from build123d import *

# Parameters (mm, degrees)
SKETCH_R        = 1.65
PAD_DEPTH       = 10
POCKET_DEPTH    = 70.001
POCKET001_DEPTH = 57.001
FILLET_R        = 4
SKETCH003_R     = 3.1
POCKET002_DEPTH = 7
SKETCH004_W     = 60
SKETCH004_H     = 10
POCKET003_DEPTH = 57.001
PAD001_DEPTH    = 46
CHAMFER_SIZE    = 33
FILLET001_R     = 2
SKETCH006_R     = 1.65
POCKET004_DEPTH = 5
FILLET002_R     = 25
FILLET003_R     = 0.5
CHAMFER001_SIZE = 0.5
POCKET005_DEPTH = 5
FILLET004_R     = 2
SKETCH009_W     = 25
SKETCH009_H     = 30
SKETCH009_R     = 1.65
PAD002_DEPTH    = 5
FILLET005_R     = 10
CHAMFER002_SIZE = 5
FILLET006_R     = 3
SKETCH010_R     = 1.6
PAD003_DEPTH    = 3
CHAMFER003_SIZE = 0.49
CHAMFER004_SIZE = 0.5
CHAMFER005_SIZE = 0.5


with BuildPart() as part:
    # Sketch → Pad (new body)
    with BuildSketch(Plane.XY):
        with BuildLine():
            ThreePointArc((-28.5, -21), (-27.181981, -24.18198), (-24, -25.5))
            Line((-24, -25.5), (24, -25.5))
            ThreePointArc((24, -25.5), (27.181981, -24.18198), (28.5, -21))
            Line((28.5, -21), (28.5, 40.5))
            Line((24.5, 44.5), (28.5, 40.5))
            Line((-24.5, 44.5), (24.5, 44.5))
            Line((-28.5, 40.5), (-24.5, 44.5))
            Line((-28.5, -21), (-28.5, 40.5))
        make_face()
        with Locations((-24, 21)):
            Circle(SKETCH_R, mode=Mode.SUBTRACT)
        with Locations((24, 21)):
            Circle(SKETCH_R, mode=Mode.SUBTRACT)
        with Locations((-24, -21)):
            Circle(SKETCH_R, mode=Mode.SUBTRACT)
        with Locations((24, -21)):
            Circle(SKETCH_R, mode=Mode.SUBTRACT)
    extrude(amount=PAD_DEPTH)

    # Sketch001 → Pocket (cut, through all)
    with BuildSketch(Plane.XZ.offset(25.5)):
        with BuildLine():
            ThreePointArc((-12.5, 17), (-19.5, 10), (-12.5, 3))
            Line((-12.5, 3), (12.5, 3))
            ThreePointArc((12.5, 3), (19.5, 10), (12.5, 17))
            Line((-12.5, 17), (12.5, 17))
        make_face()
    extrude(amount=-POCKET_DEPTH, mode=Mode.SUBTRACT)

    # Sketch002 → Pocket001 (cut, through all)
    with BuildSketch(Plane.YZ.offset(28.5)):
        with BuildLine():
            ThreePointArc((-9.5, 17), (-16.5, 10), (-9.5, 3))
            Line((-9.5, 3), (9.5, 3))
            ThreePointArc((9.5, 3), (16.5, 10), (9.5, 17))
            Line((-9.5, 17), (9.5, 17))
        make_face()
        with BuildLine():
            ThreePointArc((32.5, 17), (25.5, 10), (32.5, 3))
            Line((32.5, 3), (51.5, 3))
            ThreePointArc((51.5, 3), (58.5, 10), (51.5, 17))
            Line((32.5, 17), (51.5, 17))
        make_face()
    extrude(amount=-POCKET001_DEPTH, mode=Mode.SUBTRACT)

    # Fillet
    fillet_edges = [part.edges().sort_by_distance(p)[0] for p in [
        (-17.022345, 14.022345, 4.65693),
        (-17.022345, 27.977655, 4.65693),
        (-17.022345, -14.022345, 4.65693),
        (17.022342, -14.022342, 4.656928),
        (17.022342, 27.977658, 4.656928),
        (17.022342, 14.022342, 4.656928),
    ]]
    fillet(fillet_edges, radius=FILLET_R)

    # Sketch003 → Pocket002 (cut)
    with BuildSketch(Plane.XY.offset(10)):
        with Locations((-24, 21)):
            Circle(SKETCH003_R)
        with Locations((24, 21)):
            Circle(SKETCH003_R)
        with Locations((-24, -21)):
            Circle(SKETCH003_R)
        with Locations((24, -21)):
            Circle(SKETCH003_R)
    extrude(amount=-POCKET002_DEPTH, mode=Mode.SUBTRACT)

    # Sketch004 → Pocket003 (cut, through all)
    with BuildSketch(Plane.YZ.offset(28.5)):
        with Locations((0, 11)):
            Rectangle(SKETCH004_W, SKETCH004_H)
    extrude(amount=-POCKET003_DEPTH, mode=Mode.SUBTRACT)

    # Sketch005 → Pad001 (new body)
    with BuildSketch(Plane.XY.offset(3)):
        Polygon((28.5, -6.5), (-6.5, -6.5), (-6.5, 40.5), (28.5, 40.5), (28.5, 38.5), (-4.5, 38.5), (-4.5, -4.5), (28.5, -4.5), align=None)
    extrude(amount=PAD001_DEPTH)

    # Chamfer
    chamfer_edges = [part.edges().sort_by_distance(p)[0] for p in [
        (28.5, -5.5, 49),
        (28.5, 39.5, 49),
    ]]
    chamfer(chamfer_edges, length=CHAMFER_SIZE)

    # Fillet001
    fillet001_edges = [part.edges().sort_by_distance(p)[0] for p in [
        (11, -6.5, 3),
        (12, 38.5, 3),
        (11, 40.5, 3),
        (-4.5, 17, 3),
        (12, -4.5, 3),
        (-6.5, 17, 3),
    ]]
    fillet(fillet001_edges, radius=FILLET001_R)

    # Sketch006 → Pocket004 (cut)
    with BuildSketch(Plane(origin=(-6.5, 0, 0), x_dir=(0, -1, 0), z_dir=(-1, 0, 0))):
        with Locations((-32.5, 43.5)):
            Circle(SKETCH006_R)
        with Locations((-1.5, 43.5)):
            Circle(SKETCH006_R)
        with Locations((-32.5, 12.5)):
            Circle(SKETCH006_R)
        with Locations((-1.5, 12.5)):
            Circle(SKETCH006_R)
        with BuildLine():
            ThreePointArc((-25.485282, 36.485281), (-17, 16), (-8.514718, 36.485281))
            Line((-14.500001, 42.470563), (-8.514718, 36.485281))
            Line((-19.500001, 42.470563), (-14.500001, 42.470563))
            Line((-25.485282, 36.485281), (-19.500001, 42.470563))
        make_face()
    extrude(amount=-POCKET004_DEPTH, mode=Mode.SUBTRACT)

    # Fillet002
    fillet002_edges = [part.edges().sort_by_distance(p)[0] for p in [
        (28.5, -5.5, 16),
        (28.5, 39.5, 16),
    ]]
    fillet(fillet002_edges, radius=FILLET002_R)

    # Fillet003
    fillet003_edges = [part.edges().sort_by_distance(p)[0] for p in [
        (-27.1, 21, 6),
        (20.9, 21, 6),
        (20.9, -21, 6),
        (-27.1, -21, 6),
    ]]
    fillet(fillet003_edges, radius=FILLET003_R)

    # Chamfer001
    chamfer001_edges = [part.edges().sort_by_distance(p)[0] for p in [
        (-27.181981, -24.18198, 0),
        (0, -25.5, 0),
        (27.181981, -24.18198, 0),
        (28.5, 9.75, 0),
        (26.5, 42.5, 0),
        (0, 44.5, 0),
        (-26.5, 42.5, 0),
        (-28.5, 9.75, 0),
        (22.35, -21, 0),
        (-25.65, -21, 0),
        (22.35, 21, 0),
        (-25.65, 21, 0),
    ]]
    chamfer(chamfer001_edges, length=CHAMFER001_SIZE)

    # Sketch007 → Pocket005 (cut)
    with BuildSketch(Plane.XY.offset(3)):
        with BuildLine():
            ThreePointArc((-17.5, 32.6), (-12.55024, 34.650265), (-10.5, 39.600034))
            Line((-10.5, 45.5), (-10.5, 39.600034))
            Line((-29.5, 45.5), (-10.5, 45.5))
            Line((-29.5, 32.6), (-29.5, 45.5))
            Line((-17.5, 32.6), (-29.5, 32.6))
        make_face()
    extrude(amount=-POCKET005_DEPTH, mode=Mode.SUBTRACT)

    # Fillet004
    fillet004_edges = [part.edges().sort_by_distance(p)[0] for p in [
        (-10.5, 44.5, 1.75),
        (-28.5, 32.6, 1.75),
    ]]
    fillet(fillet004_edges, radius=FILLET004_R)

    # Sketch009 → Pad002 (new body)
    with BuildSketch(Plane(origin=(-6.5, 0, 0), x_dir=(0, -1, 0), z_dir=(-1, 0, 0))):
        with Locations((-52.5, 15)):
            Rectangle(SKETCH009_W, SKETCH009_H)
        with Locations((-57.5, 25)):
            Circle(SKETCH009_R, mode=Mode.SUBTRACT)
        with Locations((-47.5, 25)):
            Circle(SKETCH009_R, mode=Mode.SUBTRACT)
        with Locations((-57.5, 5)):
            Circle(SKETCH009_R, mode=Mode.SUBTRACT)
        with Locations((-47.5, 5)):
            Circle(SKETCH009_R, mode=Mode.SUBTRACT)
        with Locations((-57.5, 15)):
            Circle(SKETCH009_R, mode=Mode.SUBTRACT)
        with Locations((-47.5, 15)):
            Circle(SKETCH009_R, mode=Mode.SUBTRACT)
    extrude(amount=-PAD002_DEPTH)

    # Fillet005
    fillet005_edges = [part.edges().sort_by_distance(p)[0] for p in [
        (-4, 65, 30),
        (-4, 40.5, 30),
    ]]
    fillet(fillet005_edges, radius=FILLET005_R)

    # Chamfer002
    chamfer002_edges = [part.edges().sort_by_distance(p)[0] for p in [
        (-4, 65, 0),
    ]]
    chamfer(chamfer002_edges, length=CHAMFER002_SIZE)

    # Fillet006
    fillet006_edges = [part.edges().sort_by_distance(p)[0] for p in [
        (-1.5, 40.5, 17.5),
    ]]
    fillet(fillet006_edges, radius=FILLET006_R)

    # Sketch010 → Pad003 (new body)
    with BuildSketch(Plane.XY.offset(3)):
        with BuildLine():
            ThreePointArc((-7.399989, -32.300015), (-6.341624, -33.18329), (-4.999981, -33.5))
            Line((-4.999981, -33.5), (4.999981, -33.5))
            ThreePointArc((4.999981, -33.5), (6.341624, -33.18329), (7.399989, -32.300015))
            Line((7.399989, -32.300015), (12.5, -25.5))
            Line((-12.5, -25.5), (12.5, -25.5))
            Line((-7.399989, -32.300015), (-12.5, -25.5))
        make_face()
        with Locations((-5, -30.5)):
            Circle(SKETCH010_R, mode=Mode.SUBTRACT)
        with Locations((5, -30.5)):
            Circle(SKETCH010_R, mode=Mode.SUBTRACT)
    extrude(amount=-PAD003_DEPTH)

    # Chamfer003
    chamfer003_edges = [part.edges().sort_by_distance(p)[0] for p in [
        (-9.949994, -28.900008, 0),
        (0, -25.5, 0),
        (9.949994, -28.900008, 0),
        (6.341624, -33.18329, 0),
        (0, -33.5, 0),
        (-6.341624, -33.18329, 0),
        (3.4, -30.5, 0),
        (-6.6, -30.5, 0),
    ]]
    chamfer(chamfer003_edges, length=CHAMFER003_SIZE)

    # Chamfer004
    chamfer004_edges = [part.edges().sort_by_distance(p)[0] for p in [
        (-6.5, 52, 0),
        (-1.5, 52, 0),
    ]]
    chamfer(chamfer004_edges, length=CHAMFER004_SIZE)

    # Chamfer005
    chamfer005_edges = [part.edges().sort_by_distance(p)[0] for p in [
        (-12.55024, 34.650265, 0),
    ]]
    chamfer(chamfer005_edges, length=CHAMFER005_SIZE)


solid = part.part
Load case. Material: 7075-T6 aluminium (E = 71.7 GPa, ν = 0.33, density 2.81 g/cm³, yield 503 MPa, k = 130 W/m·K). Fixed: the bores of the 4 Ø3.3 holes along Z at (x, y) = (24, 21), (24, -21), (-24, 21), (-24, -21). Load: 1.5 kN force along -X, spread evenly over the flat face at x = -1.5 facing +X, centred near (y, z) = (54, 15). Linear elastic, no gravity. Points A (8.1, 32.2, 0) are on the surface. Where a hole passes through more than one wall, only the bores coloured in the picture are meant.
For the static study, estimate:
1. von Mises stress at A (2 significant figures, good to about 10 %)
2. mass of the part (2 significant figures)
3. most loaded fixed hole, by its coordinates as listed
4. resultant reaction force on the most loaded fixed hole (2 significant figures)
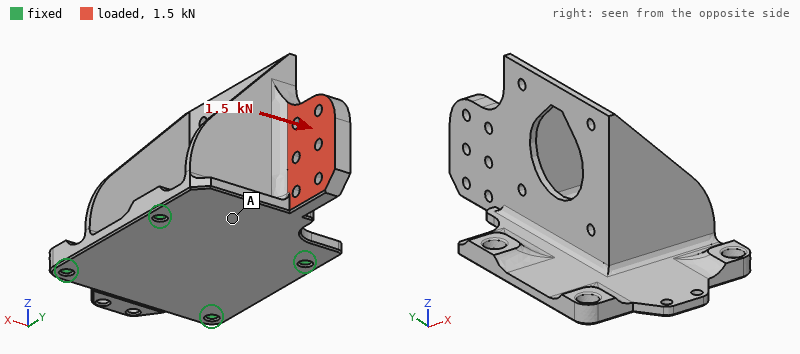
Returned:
25 MPa
67 g
(24, 21)
1.5 kN
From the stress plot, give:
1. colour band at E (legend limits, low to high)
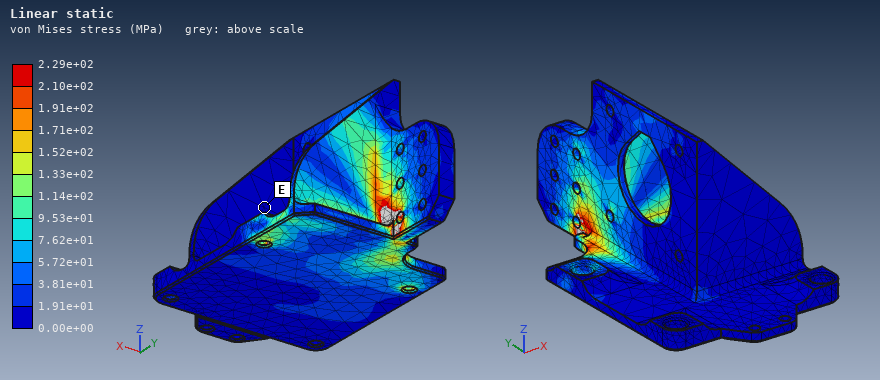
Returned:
0.00e+00 to 1.91e+01 MPa
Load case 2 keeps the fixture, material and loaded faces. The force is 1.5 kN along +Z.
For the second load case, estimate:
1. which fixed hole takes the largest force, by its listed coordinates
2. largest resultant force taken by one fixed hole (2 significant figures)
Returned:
(-24, 21)
1.4 kN
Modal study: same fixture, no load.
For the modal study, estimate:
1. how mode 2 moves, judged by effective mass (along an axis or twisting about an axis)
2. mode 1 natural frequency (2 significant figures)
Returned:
along X
1700 Hz
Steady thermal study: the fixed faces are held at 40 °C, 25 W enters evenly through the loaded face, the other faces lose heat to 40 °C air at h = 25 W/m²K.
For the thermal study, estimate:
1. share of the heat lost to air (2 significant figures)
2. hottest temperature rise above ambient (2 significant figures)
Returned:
25 %
53 K
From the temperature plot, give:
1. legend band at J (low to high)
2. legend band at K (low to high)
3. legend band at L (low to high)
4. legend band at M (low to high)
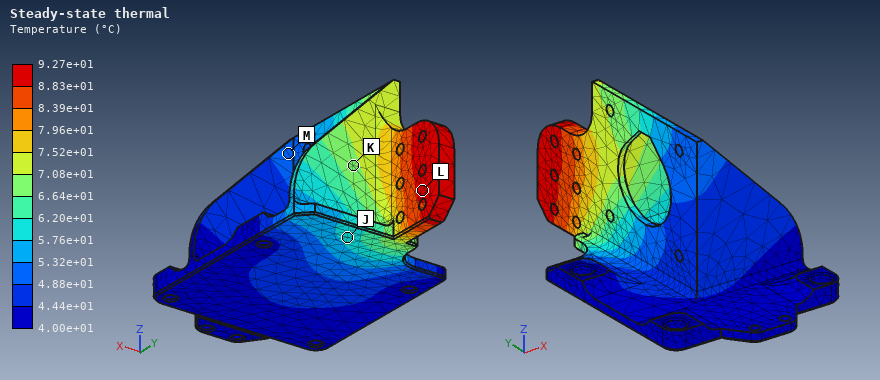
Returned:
5.76e+01 to 6.20e+01 °C
6.64e+01 to 7.08e+01 °C
8.83e+01 to 9.27e+01 °C
4.88e+01 to 5.32e+01 °C
